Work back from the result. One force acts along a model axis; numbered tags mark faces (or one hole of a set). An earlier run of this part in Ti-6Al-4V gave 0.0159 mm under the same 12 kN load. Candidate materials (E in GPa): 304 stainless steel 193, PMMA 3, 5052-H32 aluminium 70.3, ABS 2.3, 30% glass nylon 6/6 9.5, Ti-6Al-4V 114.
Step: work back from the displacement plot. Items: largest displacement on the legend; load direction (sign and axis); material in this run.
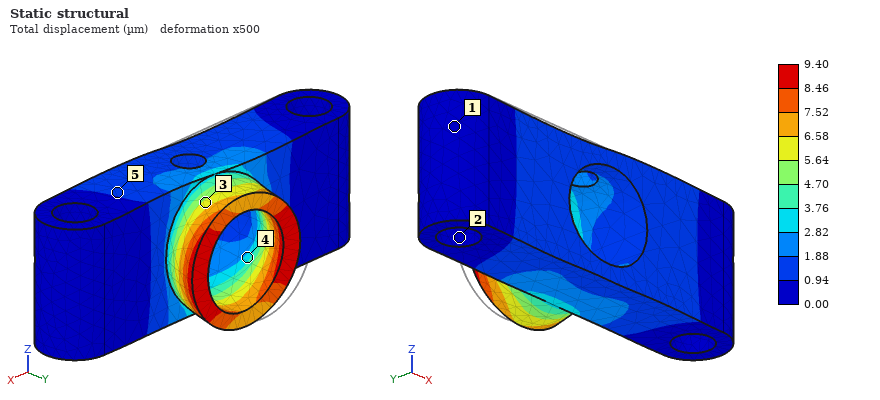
9.40 µm
+X
304 stainless steel
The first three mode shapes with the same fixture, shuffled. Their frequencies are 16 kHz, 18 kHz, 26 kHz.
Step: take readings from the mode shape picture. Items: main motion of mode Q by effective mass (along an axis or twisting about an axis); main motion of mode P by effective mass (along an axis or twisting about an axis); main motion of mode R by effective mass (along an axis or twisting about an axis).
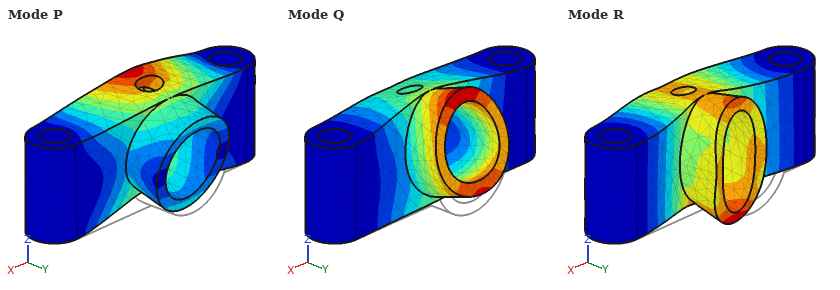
along Z
along Z
along Y
